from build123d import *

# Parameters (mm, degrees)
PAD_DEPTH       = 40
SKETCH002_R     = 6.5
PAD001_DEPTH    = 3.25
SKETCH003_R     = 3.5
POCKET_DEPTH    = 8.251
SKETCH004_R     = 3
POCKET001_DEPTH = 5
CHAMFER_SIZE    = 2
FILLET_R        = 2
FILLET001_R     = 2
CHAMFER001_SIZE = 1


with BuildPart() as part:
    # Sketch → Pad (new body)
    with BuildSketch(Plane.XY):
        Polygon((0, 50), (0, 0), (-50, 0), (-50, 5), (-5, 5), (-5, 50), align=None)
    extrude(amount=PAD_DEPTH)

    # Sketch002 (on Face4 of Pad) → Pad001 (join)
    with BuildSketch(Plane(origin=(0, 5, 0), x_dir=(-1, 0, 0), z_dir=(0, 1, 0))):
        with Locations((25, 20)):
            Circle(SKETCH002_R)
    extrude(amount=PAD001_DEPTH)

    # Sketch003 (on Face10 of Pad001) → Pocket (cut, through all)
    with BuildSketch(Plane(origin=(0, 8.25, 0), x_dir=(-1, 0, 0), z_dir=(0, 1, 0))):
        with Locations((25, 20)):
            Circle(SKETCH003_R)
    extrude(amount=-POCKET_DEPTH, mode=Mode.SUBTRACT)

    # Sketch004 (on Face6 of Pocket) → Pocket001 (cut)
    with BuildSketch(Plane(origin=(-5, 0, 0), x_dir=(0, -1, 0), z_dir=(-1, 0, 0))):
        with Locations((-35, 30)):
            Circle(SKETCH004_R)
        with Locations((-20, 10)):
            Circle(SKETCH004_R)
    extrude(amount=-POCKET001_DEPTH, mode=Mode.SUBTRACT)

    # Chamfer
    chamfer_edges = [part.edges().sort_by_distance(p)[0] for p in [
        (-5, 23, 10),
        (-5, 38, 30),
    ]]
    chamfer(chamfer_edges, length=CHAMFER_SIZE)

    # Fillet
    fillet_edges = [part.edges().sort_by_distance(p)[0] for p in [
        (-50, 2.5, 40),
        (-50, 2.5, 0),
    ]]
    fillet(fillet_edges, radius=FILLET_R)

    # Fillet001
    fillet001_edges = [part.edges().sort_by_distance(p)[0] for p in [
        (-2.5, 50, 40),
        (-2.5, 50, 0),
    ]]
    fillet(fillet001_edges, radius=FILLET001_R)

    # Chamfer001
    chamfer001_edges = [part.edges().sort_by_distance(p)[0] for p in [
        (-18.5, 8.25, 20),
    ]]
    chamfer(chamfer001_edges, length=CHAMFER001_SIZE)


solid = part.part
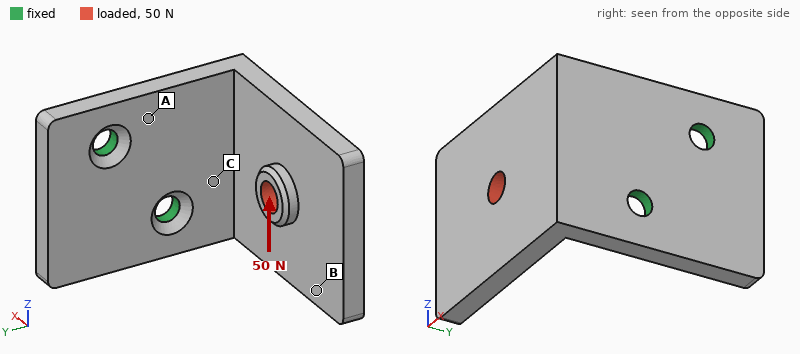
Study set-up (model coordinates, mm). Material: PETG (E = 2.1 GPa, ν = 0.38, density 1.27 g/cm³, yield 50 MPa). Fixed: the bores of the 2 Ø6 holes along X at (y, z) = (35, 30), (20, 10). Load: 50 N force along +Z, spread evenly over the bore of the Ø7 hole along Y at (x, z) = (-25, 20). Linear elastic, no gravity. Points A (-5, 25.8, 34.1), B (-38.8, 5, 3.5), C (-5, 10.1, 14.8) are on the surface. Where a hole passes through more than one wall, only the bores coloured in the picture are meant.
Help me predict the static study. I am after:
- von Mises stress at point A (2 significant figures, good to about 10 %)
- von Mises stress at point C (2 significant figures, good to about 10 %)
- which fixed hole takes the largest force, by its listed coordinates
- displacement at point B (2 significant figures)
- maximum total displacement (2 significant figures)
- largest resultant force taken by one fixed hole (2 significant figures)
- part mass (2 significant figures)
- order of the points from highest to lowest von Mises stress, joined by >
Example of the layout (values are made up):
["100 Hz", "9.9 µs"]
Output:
["2.8 MPa", "4.7 MPa", "(20, 10)", "0.55 mm", "0.84 mm", "61 N", "24 g", "C > A > B"]
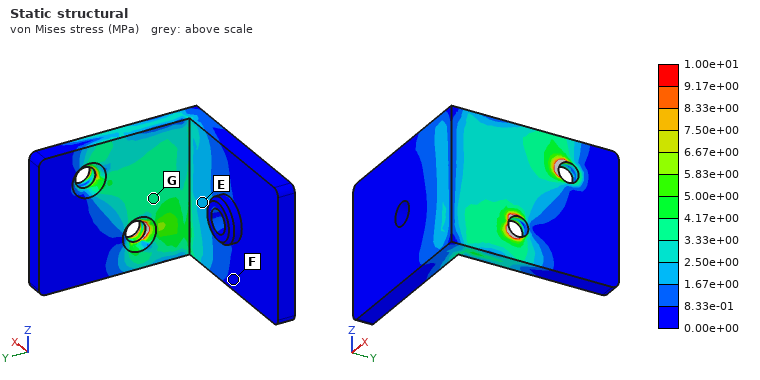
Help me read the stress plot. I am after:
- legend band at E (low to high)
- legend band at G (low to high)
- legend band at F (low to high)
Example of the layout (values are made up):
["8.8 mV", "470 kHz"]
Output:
["1.67e+00 to 2.50e+00 MPa", "3.33e+00 to 4.17e+00 MPa", "0.00e+00 to 8.33e-01 MPa"]
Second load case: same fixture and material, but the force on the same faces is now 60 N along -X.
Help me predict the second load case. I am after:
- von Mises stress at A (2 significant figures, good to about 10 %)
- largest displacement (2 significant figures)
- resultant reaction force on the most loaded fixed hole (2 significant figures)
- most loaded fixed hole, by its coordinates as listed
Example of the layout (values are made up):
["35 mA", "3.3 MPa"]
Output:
["2.9 MPa", "0.77 mm", "57 N", "(20, 10)"]
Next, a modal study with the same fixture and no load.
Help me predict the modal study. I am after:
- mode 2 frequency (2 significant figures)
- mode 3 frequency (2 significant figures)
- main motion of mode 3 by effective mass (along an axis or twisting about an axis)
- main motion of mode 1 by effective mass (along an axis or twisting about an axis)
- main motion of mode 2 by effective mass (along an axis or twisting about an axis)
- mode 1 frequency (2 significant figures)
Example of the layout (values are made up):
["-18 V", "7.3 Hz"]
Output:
["430 Hz", "1000 Hz", "along X", "along Y", "along Z", "270 Hz"]
